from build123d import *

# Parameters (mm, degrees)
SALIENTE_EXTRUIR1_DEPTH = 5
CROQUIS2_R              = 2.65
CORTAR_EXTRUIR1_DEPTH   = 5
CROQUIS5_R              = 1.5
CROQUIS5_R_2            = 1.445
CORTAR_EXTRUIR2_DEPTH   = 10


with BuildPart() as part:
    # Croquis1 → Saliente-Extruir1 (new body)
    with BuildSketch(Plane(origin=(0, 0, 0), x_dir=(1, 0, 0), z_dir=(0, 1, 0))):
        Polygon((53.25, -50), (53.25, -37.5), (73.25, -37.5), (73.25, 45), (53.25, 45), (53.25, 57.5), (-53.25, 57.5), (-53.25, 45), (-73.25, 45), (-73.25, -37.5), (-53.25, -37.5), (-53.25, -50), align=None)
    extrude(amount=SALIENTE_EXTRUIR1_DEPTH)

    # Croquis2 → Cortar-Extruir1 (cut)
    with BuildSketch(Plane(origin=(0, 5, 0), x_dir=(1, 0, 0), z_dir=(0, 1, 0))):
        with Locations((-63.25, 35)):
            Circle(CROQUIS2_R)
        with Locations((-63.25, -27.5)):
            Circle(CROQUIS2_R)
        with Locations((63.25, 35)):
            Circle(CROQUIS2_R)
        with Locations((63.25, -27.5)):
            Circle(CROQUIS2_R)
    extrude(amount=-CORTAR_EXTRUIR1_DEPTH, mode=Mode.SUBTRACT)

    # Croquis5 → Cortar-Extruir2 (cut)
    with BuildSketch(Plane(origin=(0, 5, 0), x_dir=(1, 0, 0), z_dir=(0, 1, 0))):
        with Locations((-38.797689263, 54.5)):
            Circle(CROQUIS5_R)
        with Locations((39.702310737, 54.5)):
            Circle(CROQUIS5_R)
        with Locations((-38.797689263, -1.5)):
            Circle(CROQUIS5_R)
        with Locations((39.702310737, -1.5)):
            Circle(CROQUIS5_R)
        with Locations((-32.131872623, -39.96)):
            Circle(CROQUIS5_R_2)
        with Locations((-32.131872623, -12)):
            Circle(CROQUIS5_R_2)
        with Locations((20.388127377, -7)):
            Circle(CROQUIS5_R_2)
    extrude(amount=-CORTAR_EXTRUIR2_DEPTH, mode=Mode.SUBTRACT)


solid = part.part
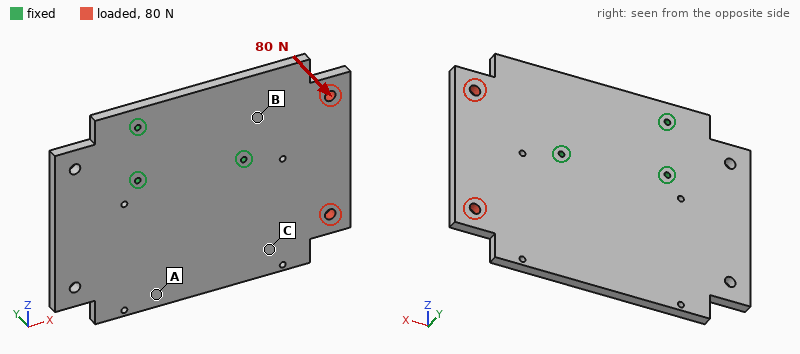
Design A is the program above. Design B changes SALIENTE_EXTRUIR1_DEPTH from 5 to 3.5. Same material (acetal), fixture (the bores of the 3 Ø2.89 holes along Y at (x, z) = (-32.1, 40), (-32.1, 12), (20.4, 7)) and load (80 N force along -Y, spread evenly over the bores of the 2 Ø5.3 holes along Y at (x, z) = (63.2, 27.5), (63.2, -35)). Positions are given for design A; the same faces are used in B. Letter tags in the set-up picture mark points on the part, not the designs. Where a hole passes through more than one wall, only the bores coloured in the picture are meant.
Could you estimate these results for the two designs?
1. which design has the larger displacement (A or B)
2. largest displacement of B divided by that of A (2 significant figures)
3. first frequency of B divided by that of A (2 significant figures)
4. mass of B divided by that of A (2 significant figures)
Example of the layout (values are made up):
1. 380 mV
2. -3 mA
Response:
1. B
2. 2.8
3. 0.72
4. 0.70
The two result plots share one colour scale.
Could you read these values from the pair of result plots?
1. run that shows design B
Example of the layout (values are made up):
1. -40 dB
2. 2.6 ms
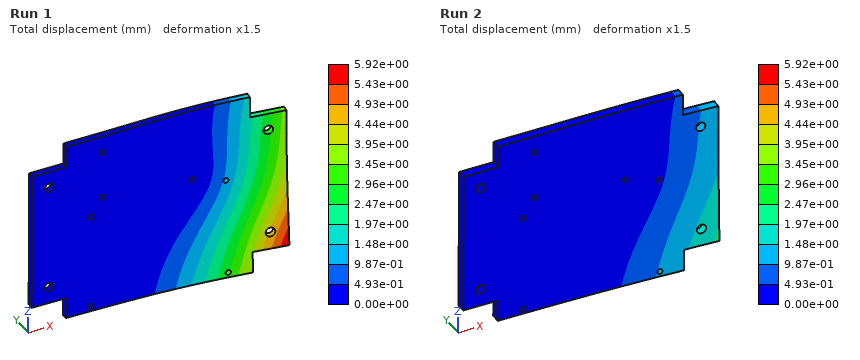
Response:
1. Run 1
